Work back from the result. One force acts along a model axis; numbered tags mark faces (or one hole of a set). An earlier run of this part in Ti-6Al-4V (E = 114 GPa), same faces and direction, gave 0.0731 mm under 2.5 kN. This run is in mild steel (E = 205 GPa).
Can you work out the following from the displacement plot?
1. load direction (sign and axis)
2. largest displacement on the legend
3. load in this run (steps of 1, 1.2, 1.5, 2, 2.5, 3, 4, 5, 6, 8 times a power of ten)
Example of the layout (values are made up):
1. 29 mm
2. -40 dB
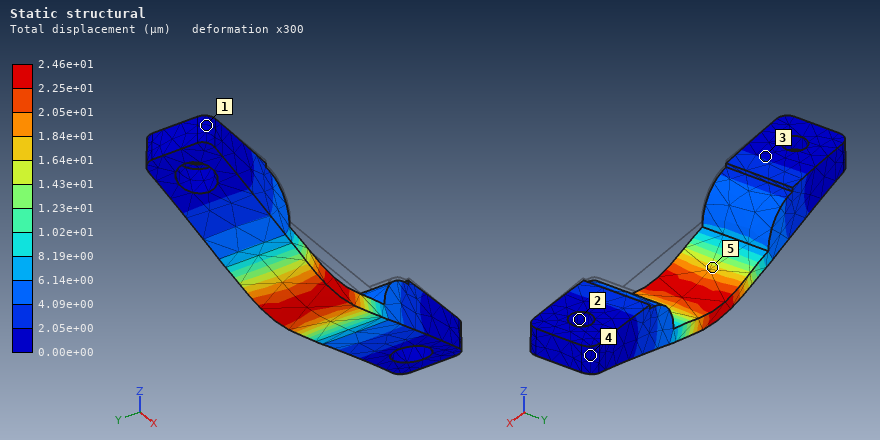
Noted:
1. -Z
2. 2.46e+01 µm
3. 1.5 kN
